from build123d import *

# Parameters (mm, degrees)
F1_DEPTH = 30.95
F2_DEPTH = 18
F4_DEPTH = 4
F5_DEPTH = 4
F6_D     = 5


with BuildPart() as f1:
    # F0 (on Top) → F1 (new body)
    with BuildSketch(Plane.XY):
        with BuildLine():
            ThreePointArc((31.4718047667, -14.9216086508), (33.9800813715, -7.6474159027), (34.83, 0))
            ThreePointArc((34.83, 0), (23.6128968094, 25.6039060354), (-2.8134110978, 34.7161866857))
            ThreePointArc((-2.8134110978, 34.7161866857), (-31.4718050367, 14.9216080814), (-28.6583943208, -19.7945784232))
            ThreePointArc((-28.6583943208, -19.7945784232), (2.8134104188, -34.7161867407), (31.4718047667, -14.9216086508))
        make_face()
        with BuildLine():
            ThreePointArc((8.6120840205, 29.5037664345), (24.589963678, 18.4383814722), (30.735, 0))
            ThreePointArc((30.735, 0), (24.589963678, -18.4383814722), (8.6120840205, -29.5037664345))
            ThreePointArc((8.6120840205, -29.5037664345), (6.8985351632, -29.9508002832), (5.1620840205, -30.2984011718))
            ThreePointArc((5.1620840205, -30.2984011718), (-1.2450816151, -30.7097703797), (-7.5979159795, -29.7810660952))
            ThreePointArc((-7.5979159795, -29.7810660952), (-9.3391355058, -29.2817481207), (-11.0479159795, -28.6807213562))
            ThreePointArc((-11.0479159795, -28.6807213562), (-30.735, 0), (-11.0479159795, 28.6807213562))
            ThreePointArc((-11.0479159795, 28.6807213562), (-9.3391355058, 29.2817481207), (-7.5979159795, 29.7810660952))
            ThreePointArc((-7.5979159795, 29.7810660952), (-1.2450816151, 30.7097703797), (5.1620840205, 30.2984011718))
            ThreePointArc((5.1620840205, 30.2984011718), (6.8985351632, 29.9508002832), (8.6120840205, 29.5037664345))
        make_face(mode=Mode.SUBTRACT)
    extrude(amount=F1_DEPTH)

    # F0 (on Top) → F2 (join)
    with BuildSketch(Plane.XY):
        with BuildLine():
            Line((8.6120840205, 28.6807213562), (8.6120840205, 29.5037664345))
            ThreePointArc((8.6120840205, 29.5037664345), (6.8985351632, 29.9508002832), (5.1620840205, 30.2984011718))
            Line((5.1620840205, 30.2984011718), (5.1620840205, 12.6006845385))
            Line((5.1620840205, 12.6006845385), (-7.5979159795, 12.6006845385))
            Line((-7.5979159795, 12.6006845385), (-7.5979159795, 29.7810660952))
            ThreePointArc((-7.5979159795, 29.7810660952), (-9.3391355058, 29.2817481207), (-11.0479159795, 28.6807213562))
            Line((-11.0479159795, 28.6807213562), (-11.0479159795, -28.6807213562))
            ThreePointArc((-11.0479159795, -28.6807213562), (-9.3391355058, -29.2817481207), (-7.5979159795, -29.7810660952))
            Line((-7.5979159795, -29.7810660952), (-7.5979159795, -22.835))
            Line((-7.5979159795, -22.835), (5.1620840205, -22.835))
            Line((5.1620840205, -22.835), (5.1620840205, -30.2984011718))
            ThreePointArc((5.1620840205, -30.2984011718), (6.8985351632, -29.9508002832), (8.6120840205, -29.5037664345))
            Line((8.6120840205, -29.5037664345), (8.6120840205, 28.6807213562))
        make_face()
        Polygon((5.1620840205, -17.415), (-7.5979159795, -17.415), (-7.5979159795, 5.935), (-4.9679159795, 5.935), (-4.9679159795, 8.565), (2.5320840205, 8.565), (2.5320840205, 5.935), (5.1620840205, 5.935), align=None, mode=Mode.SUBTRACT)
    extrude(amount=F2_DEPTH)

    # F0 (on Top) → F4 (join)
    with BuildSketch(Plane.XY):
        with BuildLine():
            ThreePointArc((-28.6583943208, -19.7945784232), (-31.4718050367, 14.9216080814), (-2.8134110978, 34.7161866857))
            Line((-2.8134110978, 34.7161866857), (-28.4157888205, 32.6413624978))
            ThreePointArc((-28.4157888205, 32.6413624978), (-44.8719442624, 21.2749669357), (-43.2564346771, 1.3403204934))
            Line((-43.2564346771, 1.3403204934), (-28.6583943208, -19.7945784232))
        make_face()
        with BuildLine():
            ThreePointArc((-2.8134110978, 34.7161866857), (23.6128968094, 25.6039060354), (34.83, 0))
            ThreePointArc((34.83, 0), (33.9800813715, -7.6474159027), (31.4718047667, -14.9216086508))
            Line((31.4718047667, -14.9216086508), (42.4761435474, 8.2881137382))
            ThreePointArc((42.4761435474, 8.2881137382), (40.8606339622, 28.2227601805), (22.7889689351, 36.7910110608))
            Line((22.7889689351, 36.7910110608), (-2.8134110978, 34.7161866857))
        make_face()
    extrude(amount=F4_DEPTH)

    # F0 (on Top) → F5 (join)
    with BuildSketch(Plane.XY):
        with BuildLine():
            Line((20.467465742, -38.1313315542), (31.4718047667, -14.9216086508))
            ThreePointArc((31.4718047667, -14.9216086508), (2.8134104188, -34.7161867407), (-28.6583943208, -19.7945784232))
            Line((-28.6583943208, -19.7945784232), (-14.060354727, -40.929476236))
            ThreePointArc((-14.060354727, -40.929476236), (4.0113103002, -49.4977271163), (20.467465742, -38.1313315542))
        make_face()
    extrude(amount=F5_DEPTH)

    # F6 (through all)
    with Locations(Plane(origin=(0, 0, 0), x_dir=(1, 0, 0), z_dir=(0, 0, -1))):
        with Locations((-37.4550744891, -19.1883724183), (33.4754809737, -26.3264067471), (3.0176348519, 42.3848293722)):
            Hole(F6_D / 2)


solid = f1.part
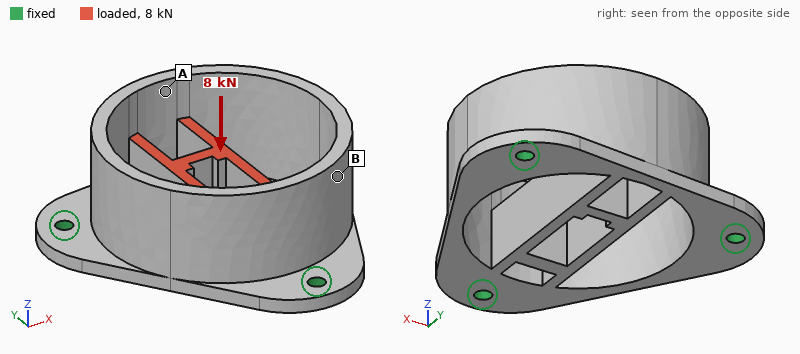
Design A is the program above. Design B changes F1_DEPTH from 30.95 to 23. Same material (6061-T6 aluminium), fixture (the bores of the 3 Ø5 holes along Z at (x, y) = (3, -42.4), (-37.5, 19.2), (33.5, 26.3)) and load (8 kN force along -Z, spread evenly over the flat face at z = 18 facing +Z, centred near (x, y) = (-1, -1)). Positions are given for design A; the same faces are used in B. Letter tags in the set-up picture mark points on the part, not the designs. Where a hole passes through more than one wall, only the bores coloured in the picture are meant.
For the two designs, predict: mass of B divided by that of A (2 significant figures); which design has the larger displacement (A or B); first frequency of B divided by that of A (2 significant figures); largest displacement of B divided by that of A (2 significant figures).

0.84
B
1.1
1.1
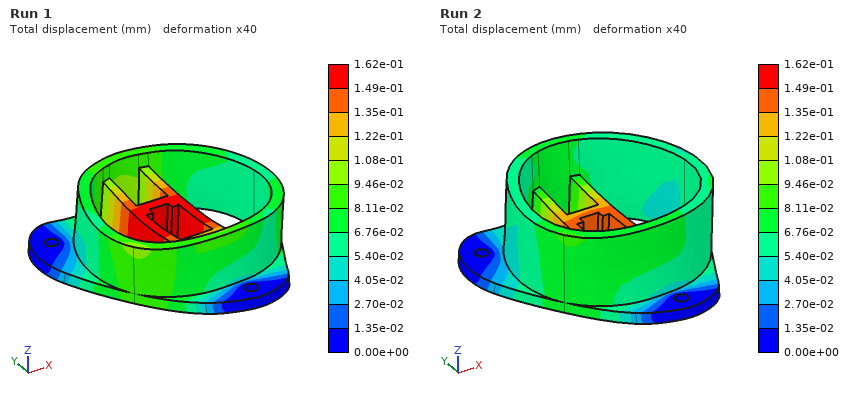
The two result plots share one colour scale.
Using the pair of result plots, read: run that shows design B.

Run 1
